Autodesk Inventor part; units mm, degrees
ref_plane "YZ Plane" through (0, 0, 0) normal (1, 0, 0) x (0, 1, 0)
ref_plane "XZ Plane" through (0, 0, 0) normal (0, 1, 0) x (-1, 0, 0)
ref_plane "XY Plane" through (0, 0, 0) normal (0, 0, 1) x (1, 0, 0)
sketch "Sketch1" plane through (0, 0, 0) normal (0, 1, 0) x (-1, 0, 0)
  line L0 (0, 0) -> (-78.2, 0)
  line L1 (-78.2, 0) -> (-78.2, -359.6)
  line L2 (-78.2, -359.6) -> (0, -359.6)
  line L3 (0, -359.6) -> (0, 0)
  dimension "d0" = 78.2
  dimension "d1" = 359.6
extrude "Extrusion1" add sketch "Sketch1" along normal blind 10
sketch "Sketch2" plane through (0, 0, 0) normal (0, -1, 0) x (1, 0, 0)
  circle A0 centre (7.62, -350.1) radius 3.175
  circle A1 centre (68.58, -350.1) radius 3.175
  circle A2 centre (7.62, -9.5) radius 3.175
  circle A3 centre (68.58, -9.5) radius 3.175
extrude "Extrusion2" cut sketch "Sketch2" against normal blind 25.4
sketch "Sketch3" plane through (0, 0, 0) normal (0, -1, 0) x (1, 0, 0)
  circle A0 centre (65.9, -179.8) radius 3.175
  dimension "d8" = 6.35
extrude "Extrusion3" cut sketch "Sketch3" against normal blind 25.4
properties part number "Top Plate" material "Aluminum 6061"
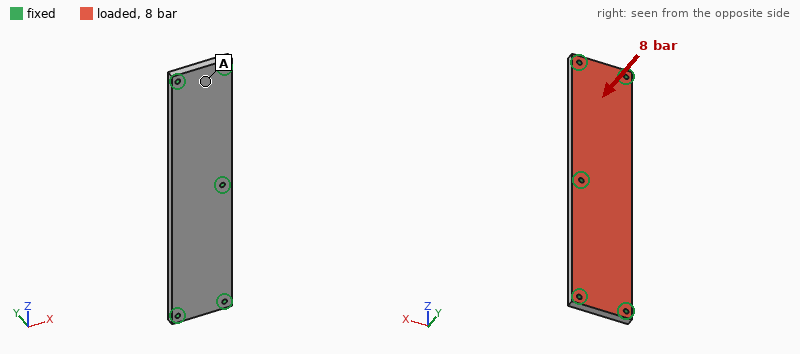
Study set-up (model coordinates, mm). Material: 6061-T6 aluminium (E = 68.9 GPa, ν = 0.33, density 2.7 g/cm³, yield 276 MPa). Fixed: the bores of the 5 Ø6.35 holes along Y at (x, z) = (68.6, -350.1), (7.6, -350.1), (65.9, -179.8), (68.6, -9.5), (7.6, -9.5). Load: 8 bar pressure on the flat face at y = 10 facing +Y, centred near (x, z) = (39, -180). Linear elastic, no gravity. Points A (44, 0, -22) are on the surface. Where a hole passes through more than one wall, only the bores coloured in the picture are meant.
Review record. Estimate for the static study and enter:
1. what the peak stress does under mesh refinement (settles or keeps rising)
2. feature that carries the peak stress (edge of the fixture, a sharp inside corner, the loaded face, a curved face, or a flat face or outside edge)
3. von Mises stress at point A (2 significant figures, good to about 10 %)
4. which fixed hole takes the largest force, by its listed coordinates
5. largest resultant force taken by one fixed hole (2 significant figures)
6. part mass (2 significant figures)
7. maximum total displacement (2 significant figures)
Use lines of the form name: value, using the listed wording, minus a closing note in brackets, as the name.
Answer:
what the peak stress does under mesh refinement: keeps rising
feature that carries the peak stress: edge of the fixture
von Mises stress at point A: 41 MPa
which fixed hole takes the largest force, by its listed coordinates: (65.9, -179.8)
largest resultant force taken by one fixed hole: 11 kN
part mass: 750 g
maximum total displacement: 0.73 mm
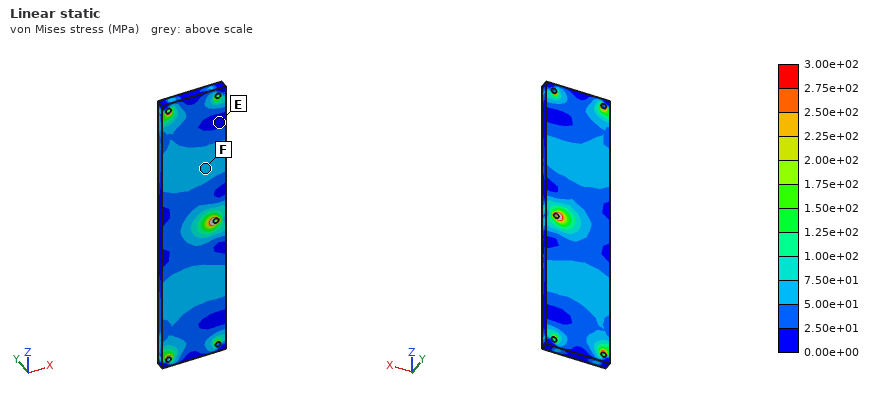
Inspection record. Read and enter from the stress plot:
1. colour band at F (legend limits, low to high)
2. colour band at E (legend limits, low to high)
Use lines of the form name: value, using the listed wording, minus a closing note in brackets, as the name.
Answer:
colour band at F: 5.00e+01 to 7.50e+01 MPa
colour band at E: 0.00e+00 to 2.50e+01 MPa
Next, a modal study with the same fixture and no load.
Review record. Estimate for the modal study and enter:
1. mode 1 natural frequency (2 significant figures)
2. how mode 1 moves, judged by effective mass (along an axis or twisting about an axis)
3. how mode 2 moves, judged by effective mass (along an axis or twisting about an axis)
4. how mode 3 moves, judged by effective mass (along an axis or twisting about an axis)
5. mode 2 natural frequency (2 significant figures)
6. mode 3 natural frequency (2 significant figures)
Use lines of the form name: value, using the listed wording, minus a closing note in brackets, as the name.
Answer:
mode 1 natural frequency: 1300 Hz
how mode 1 moves, judged by effective mass: along Y
how mode 2 moves, judged by effective mass: twisting about X
how mode 3 moves, judged by effective mass: along Y
mode 2 natural frequency: 1400 Hz
mode 3 natural frequency: 2100 Hz
